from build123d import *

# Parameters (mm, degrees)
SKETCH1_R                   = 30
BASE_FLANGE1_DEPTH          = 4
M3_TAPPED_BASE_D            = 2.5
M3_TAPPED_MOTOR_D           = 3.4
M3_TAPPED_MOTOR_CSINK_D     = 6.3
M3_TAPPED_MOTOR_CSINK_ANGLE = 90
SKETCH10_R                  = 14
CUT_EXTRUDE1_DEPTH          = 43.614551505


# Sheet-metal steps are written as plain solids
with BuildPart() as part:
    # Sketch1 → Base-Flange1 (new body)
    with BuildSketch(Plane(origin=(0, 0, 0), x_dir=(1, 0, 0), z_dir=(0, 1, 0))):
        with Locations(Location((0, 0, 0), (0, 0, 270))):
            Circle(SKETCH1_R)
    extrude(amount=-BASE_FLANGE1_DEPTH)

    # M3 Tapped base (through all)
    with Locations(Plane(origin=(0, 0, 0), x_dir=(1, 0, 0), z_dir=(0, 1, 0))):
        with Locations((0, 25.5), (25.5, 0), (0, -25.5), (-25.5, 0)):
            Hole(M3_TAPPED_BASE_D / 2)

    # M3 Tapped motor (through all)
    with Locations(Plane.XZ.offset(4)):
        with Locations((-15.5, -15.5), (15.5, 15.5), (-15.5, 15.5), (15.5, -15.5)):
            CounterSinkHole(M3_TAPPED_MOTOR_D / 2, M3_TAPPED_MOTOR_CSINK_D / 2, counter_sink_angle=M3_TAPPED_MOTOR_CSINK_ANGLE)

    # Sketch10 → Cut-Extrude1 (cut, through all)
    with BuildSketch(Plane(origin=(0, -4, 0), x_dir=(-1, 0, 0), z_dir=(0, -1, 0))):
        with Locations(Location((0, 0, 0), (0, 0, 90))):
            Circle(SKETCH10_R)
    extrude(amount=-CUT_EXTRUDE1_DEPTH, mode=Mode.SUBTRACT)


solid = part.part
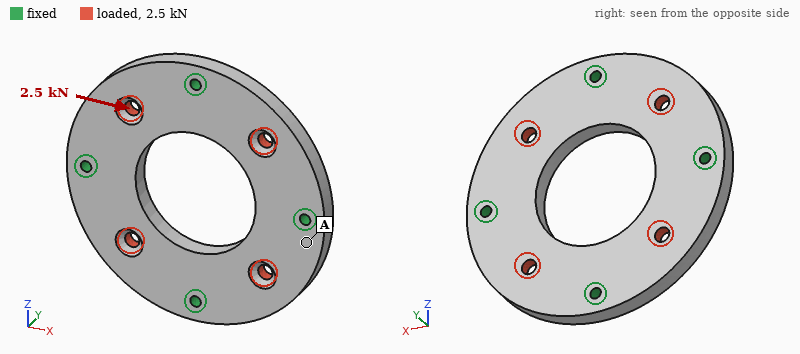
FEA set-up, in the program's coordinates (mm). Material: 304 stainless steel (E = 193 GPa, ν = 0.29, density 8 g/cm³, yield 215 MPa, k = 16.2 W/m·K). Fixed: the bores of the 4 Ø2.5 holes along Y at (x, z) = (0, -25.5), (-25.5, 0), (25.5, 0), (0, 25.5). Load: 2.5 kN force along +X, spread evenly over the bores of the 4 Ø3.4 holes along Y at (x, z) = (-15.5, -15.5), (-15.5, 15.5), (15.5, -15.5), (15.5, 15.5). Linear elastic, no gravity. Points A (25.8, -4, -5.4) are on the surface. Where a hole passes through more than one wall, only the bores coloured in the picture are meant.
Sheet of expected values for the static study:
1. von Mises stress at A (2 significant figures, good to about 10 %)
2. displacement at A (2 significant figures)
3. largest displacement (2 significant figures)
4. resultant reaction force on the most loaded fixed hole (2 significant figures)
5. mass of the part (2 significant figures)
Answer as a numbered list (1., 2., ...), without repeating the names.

1. 6.3 MPa
2. 0.50 µm
3. 2.1 µm
4. 780 N
5. 69 g
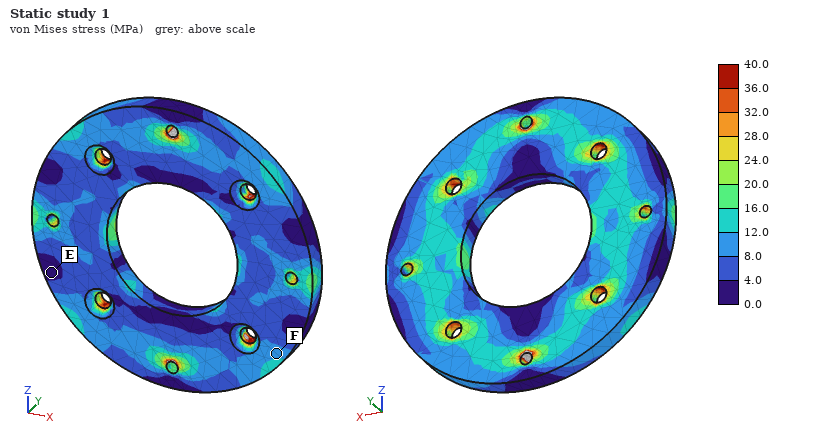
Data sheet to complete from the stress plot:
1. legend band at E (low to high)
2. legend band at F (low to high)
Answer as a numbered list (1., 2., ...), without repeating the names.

1. 0.0 to 4.0 MPa
2. 8.0 to 12.0 MPa
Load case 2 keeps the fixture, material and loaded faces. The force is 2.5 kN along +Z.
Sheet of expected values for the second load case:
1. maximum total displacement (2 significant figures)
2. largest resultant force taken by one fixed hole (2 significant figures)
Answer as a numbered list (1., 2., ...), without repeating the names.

1. 2.1 µm
2. 780 N
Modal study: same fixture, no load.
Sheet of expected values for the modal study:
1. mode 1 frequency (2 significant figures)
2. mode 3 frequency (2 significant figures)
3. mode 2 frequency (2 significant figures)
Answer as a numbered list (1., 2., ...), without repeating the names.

1. 10 kHz
2. 11 kHz
3. 11 kHz
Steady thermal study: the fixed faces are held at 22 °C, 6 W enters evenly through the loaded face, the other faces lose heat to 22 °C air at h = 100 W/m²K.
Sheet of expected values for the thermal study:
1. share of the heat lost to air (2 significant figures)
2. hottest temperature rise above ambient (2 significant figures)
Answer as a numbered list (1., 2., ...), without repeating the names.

1. 51 %
2. 14 K
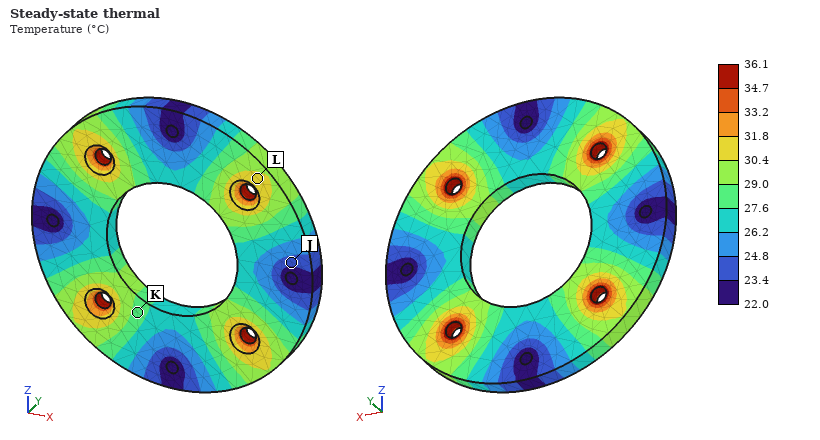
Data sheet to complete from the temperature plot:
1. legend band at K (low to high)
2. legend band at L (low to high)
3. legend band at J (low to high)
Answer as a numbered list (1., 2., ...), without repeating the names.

1. 27.6 to 29.0 °C
2. 30.4 to 31.8 °C
3. 23.4 to 24.8 °C
